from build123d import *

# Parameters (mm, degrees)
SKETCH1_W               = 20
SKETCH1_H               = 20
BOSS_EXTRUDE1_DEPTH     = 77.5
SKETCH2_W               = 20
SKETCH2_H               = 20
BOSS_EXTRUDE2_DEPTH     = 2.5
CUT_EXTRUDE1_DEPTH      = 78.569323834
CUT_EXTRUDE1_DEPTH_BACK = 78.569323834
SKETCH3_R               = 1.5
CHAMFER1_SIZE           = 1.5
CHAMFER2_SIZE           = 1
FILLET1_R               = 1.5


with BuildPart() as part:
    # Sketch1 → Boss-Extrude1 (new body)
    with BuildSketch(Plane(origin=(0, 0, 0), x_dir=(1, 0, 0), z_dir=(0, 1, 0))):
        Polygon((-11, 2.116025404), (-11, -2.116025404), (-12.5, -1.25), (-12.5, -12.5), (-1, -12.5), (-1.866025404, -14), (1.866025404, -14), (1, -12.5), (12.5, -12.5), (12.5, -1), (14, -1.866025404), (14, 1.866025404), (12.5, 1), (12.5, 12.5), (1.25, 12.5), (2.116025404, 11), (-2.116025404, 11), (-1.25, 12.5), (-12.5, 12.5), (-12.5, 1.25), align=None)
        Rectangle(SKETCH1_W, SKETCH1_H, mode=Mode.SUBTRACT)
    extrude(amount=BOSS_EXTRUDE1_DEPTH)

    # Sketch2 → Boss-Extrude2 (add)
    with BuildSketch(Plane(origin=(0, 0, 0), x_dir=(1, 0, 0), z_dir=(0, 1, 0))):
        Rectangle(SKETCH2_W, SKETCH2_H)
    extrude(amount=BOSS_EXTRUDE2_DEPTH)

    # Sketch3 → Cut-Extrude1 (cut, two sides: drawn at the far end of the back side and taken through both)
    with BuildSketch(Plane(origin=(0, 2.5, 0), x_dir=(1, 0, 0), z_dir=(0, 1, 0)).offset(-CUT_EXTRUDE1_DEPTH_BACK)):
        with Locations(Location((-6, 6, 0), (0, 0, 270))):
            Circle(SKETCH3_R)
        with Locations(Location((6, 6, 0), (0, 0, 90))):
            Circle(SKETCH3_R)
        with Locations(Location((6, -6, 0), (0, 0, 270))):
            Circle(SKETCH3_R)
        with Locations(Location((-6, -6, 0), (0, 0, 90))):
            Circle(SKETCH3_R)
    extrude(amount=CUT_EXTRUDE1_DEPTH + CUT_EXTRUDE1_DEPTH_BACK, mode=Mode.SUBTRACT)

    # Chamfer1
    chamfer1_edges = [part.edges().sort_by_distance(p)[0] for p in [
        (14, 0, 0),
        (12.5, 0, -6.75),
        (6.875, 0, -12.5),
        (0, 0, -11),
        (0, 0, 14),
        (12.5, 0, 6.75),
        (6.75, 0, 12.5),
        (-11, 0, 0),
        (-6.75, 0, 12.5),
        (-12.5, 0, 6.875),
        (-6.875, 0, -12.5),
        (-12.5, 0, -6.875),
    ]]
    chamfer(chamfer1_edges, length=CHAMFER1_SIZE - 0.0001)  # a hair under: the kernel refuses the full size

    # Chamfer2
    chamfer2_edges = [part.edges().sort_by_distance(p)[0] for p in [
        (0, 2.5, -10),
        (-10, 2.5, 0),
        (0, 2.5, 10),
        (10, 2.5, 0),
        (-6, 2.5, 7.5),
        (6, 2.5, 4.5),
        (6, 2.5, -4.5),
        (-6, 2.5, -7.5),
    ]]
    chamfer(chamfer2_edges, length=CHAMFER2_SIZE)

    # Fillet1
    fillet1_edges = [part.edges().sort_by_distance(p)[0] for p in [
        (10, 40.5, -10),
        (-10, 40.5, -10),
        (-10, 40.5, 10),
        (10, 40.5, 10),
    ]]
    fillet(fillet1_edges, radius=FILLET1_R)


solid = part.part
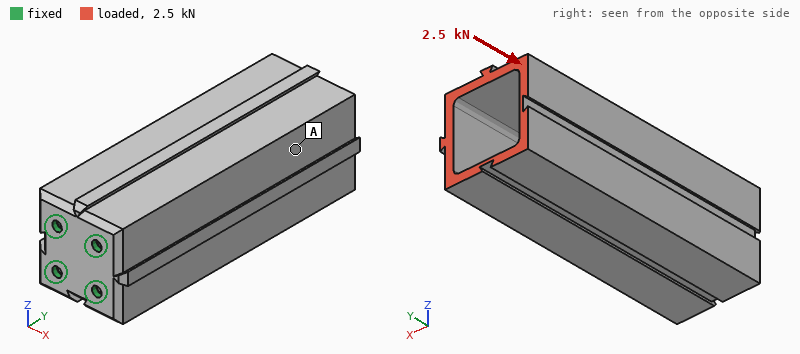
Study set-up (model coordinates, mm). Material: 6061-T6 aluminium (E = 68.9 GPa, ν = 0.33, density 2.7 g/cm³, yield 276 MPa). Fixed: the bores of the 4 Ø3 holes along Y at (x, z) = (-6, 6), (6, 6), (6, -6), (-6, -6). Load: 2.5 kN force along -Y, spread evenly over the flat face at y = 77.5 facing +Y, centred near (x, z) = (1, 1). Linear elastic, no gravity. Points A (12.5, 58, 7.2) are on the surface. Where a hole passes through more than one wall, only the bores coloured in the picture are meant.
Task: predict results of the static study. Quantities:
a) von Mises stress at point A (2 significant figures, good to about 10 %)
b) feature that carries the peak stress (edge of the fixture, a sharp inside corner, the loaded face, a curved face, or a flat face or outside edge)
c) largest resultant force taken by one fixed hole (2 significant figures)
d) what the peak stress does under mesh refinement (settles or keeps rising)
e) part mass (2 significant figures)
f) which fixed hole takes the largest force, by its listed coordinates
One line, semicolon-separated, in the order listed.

11 MPa; edge of the fixture; 750 N; keeps rising; 49 g; (6, 6)
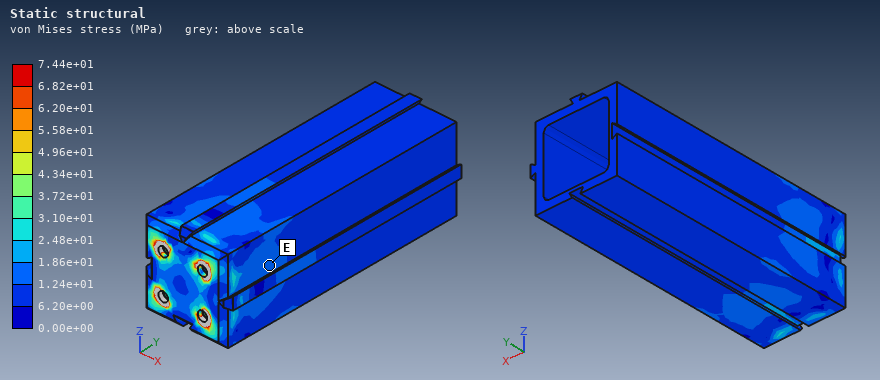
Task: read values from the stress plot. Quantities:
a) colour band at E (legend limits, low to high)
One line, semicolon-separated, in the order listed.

1.24e+01 to 1.86e+01 MPa
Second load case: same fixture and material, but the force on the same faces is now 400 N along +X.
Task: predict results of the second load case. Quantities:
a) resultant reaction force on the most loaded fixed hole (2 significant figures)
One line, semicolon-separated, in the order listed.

1.1 kN
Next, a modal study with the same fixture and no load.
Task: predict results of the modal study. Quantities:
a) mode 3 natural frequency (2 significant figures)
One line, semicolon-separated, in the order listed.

7500 Hz
